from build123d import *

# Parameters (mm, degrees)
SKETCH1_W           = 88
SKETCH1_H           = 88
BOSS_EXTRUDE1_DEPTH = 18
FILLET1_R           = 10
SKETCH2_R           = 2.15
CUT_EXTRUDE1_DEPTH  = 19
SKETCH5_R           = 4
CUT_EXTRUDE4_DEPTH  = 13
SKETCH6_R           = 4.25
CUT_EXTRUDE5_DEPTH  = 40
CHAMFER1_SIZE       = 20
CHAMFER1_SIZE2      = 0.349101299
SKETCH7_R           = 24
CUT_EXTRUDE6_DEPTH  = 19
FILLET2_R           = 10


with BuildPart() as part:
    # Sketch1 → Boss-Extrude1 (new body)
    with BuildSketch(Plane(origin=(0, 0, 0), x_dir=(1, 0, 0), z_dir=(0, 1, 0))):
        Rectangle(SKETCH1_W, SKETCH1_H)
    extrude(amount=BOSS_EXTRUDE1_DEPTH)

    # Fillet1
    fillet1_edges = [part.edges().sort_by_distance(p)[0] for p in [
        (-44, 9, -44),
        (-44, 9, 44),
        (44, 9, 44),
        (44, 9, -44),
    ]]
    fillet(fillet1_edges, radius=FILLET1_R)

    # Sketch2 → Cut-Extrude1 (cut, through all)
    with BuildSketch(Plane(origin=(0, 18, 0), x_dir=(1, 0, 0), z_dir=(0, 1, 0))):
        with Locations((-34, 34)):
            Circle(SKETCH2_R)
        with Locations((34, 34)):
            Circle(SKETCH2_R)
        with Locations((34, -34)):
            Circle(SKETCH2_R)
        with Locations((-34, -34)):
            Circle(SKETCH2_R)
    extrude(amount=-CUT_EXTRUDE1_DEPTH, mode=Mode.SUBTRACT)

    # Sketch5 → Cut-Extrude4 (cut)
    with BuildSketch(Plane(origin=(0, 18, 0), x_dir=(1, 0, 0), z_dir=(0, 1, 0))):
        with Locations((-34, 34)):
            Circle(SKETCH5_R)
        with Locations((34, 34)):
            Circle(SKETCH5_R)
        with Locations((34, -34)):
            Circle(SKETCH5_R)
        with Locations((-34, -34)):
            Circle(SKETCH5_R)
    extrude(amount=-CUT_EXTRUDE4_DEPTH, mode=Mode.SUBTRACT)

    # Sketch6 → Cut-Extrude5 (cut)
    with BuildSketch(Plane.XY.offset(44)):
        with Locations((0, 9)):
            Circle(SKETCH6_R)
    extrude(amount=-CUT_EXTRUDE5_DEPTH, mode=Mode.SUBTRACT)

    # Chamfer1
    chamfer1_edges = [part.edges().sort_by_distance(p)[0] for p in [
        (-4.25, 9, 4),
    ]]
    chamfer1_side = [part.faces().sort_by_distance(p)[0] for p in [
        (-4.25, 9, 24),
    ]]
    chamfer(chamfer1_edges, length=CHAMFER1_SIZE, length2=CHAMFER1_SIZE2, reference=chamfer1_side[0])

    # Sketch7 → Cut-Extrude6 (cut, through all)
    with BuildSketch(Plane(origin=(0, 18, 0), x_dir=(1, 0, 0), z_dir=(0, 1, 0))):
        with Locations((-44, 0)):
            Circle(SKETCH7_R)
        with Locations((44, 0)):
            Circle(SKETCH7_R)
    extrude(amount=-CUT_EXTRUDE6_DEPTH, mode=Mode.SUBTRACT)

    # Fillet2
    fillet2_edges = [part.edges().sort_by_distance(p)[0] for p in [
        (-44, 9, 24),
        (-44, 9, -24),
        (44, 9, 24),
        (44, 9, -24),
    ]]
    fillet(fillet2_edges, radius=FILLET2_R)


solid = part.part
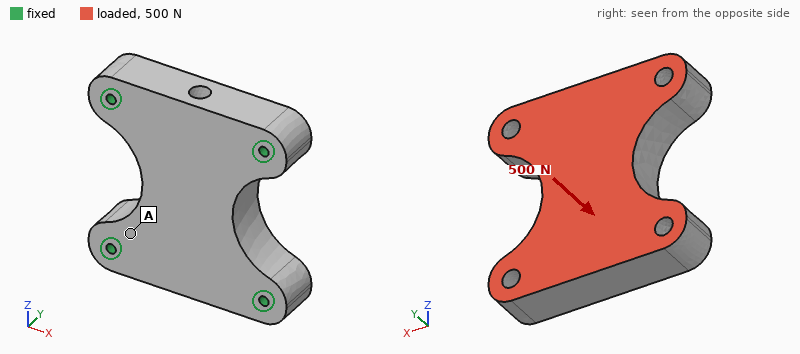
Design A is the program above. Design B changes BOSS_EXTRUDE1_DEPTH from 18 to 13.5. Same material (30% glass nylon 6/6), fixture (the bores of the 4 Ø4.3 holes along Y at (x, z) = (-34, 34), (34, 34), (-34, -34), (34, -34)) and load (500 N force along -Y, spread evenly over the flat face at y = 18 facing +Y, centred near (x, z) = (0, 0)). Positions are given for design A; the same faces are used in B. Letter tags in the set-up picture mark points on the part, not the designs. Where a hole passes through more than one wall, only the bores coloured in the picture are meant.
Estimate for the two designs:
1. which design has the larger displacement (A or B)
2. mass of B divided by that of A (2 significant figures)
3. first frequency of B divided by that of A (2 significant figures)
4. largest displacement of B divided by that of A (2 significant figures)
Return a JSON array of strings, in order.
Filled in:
["B", "0.75", "0.82", "2.0"]
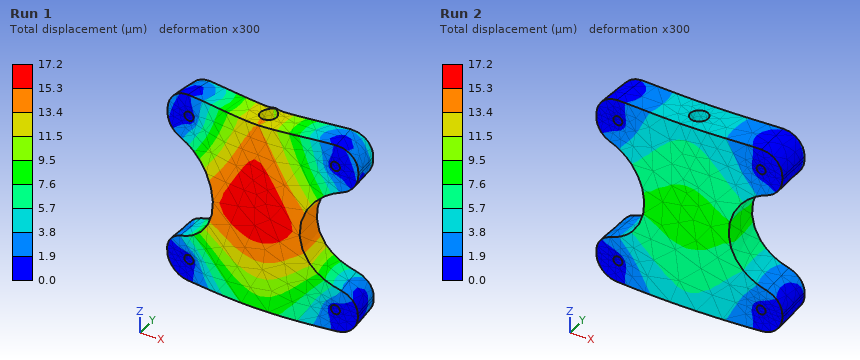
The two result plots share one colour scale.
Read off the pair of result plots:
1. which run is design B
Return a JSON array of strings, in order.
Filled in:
["Run 1"]
